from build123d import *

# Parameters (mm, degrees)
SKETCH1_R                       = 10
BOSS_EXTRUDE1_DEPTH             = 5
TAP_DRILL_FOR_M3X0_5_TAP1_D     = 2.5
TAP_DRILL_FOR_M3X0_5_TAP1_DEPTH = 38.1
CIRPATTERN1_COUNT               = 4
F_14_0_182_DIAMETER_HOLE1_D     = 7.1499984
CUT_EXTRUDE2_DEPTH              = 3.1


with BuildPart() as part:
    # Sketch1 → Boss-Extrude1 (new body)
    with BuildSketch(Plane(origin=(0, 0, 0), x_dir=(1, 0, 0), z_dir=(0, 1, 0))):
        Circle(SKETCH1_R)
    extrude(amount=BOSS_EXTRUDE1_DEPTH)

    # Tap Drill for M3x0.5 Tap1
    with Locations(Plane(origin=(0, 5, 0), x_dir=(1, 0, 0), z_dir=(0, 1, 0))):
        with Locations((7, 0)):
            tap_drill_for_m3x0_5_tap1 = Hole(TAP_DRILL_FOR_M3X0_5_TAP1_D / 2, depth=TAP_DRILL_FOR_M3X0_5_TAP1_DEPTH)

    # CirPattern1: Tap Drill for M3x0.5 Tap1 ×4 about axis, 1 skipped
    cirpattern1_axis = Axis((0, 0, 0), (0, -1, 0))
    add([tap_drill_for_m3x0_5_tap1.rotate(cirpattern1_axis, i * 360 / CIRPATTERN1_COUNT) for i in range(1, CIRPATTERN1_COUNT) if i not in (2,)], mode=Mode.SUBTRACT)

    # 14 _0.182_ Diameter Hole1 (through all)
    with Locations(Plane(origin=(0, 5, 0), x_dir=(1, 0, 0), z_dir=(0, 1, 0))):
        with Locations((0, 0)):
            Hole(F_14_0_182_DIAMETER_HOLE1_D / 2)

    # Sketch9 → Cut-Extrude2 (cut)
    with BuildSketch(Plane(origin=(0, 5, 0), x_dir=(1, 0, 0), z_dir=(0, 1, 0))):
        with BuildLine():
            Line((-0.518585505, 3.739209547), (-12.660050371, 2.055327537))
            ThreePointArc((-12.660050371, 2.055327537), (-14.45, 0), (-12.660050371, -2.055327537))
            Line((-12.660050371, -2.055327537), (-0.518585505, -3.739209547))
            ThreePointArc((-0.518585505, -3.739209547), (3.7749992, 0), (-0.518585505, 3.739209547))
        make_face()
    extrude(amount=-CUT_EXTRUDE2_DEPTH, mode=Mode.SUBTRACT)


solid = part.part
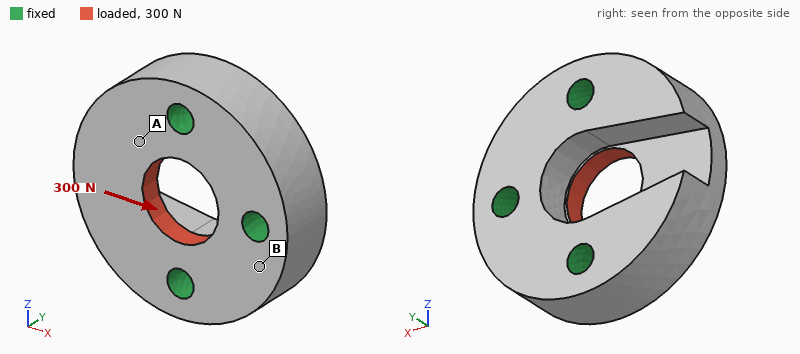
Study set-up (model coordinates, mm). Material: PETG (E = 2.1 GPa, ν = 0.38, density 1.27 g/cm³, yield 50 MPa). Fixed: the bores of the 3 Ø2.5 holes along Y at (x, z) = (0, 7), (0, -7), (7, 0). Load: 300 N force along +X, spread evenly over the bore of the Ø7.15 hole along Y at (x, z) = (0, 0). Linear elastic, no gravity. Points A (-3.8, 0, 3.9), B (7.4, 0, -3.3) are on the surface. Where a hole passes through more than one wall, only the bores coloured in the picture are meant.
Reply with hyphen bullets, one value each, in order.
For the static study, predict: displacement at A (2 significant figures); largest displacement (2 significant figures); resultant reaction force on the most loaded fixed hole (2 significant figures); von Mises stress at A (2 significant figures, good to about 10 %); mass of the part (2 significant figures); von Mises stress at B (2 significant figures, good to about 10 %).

- 22 µm
- 49 µm
- 110 N
- 7.1 MPa
- 1.5 g
- 2.7 MPa
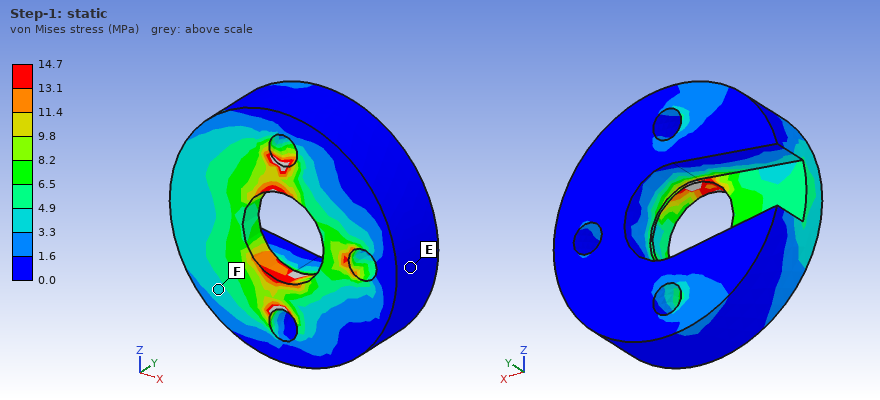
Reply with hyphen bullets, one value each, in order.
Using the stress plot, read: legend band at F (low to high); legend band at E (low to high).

- 3.3 to 4.9 MPa
- 0.0 to 1.6 MPa
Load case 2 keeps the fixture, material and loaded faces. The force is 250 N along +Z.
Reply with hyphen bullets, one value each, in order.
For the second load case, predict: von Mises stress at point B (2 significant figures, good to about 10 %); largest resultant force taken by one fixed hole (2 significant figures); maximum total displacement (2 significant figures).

- 1.6 MPa
- 100 N
- 27 µm
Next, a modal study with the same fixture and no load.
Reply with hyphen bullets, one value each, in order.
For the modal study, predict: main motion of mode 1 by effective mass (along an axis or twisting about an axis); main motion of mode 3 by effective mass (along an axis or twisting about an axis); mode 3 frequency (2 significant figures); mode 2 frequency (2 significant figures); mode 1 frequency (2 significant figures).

- along Y
- along Z
- 18 kHz
- 15 kHz
- 11 kHz
